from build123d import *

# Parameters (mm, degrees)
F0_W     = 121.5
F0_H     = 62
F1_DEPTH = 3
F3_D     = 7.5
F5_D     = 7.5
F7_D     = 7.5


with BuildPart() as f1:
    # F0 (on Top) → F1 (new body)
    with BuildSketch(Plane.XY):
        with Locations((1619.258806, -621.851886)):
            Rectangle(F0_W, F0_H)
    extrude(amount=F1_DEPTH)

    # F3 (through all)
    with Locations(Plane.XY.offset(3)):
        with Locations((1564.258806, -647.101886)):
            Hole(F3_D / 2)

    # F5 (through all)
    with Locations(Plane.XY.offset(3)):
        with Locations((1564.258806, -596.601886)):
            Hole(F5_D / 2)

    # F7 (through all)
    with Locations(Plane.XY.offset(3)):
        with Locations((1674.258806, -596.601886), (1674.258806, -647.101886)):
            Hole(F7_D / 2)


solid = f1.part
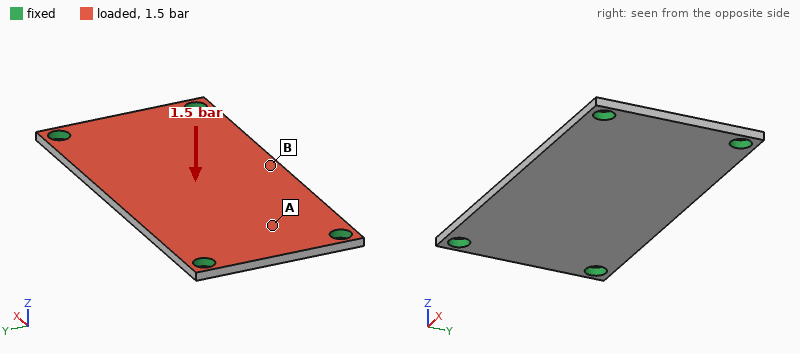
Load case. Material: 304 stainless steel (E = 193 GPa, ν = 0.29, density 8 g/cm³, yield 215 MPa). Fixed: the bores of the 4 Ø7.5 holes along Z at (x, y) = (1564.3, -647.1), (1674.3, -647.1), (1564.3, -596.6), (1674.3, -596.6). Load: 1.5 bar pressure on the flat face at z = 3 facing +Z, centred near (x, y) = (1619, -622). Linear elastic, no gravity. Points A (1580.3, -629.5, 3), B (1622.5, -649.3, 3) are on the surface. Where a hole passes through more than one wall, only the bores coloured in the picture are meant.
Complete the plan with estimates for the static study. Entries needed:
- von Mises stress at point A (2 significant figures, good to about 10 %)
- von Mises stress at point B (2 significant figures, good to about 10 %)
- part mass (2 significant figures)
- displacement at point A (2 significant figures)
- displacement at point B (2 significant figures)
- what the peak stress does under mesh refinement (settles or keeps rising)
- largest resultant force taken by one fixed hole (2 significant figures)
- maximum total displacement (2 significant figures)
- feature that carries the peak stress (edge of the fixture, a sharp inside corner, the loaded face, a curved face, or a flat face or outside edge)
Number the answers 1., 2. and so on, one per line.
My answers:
1. 24 MPa
2. 53 MPa
3. 180 g
4. 0.043 mm
5. 0.13 mm
6. keeps rising
7. 280 N
8. 0.14 mm
9. edge of the fixture
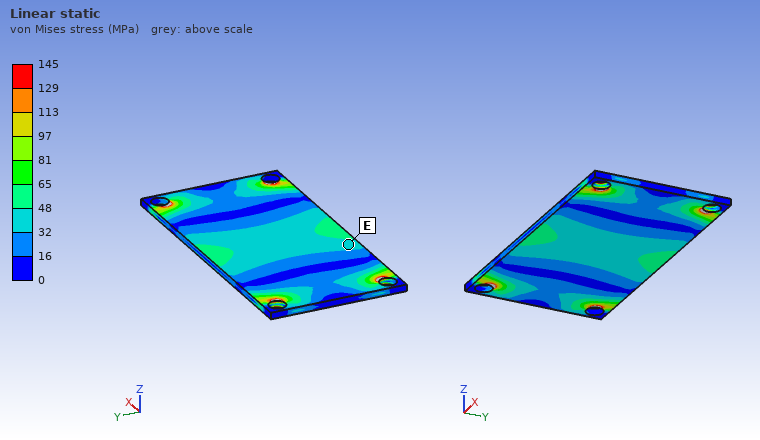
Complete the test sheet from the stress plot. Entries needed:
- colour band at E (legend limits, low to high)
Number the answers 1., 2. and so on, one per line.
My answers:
1. 32 to 48 MPa
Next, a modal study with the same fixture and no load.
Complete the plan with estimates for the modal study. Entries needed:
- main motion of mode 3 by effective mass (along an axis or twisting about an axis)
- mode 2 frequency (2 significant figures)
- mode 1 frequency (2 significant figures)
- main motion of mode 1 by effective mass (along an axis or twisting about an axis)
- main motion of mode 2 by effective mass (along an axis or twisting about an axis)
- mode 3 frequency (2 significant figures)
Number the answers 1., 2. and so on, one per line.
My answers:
1. twisting about Y
2. 2100 Hz
3. 1200 Hz
4. along Z
5. twisting about X
6. 3400 Hz
